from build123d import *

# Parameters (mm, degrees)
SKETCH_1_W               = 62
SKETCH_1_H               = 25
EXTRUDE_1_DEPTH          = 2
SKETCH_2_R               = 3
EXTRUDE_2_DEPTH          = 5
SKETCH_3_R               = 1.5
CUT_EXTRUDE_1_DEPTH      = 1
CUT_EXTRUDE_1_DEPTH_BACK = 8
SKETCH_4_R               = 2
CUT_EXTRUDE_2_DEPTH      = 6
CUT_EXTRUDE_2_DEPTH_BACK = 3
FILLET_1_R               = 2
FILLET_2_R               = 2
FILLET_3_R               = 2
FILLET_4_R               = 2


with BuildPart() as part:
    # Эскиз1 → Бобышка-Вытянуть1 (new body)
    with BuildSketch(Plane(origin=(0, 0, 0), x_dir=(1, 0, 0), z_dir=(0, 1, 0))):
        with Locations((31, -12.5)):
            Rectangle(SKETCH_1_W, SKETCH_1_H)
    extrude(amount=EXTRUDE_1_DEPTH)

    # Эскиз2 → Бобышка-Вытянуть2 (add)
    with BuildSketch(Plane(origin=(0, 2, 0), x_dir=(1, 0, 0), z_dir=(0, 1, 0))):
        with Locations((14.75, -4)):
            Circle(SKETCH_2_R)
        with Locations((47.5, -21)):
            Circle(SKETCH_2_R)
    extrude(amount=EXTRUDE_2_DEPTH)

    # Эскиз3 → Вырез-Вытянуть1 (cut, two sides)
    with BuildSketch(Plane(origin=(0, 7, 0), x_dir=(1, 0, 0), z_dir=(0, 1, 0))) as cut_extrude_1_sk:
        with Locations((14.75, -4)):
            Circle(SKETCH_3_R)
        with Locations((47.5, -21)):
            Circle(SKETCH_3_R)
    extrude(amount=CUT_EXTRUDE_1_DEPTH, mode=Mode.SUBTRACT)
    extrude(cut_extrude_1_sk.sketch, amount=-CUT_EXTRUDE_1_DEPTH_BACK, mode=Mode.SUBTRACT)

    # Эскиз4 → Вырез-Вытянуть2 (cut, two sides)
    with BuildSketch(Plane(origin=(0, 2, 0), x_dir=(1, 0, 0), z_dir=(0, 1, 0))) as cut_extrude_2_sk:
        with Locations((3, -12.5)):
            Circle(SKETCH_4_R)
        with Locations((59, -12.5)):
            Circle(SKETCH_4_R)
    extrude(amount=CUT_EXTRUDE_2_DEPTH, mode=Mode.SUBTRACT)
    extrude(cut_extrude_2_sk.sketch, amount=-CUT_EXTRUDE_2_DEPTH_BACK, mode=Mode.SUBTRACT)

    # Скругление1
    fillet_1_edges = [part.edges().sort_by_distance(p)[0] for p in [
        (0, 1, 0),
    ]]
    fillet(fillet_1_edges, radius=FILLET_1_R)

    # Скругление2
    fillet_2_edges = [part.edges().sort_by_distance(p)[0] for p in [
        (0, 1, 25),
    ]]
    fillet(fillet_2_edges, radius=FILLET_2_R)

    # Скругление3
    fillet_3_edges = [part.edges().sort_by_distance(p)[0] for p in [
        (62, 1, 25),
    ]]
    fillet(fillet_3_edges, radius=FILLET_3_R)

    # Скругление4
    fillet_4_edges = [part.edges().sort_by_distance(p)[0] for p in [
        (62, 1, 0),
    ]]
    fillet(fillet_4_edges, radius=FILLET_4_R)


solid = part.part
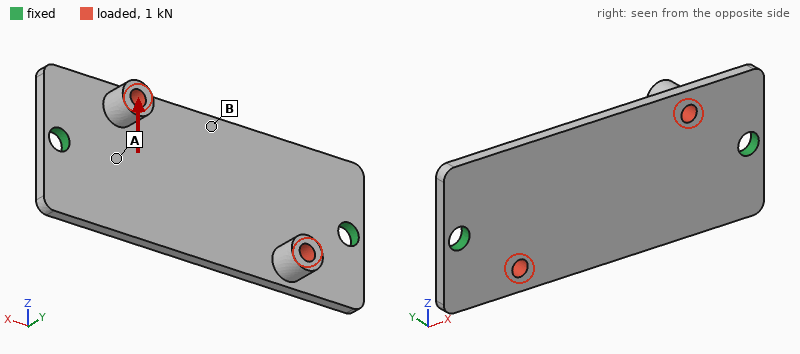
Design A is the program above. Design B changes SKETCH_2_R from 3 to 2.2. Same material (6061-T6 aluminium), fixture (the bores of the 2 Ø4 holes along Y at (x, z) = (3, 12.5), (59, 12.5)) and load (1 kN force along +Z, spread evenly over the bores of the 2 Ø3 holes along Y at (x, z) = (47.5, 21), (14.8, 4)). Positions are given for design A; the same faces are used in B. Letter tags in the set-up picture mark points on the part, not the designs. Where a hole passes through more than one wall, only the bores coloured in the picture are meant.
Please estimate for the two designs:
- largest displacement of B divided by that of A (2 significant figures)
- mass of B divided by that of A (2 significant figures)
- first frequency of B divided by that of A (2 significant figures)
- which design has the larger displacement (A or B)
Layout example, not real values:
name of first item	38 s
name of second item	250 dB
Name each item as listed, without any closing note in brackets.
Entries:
largest displacement of B divided by that of A	1.1
mass of B divided by that of A	0.96
first frequency of B divided by that of A	1.0
which design has the larger displacement	B
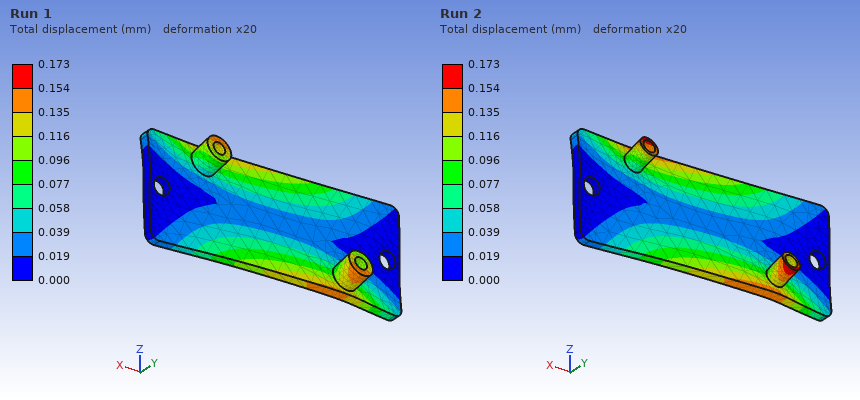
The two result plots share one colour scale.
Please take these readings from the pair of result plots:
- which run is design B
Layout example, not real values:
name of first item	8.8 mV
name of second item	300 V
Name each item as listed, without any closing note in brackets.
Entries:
which run is design B	Run 2
